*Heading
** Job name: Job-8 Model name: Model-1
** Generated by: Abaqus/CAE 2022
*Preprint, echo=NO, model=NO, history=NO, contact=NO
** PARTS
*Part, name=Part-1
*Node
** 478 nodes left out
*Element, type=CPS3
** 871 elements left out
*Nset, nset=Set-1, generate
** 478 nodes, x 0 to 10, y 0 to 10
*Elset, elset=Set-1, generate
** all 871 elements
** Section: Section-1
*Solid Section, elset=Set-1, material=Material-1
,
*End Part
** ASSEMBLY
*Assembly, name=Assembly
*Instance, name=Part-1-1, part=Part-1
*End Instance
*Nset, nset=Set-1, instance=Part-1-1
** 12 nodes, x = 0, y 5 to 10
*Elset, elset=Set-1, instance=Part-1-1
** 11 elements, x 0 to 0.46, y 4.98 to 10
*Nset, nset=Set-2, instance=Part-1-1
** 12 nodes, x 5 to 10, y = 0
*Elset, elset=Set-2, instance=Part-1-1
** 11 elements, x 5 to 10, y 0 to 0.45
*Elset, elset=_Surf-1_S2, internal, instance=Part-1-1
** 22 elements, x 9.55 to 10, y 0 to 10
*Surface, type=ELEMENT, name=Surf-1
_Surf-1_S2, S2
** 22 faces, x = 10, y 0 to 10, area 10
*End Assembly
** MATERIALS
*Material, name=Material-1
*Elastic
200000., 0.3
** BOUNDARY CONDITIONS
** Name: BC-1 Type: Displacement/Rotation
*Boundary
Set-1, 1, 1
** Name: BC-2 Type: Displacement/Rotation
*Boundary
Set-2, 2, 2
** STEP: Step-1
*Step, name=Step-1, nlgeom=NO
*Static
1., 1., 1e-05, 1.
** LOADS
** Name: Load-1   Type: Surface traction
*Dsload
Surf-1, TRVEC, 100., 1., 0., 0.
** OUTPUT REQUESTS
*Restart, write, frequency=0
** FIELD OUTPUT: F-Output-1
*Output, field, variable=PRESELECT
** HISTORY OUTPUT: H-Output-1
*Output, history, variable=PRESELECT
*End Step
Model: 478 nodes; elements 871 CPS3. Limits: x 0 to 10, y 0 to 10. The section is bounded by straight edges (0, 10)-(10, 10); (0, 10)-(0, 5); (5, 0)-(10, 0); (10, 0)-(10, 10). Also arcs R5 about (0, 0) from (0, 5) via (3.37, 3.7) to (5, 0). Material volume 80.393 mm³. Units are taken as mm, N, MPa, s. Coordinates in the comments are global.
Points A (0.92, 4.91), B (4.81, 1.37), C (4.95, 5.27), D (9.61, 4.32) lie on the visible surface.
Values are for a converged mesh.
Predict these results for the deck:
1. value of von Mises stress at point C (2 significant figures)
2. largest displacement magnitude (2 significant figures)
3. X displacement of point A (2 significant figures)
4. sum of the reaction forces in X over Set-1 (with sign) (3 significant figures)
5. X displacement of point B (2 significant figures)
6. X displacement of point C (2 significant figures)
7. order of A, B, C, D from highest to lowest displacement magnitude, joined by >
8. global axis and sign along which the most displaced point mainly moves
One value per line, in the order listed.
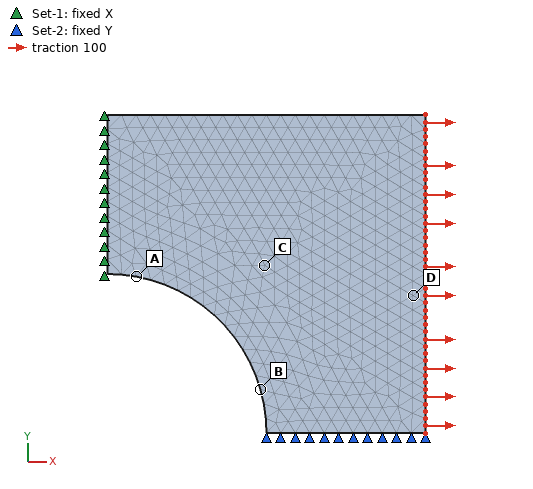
230 MPa
0.019 mm
0.0029 mm
-1000 N
0.018 mm
0.0083 mm
B > D > A > C
+X
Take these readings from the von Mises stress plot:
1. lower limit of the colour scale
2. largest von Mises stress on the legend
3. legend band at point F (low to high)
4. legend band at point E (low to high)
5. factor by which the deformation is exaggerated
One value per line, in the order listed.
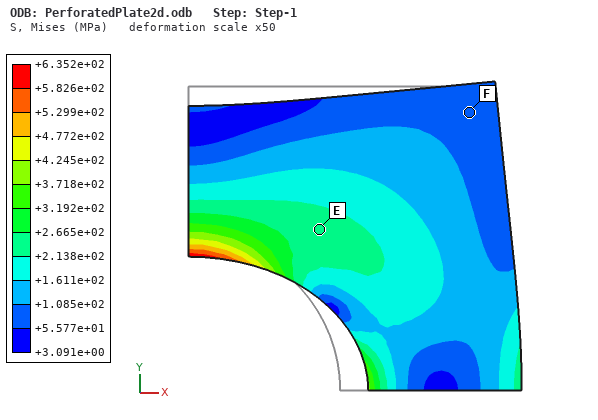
+3.091e+00 MPa
+6.352e+02 MPa
+5.577e+01 to +1.085e+02 MPa
+2.138e+02 to +2.665e+02 MPa
50
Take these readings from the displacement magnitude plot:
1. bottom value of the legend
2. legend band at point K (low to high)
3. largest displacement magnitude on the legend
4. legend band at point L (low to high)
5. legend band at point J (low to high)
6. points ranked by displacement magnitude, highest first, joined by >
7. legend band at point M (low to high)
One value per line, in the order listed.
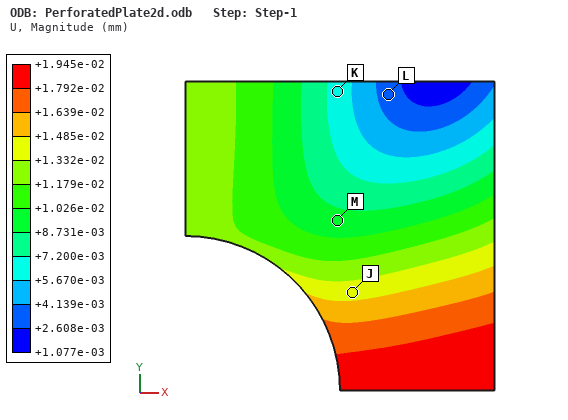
+1.077e-03 mm
+5.670e-03 to +7.200e-03 mm
+1.945e-02 mm
+2.608e-03 to +4.139e-03 mm
+1.332e-02 to +1.485e-02 mm
J > M > K > L
+8.731e-03 to +1.026e-02 mm
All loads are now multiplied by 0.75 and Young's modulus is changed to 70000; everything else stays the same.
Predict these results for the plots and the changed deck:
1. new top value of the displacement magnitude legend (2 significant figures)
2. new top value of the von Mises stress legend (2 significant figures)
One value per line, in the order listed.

0.042 mm
480 MPa
